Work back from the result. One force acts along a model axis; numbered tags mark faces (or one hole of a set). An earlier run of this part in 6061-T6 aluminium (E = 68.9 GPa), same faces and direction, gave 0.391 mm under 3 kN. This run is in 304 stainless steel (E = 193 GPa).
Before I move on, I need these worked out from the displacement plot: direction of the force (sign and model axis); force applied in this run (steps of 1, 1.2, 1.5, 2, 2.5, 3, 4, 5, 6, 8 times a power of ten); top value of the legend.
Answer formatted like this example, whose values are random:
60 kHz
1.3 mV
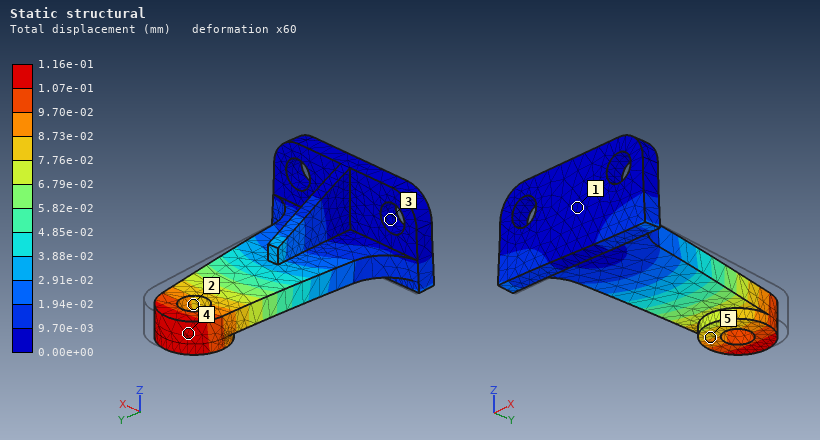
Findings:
-X
2.5 kN
1.16e-01 mm
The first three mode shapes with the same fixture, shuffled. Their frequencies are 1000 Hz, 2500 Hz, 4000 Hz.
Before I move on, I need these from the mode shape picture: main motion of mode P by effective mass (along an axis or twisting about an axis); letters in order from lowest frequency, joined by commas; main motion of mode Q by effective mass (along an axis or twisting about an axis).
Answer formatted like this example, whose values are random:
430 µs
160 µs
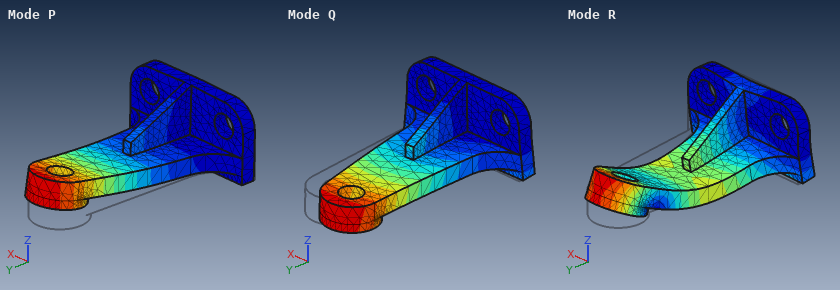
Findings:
along Z
P, Q, R
along X
